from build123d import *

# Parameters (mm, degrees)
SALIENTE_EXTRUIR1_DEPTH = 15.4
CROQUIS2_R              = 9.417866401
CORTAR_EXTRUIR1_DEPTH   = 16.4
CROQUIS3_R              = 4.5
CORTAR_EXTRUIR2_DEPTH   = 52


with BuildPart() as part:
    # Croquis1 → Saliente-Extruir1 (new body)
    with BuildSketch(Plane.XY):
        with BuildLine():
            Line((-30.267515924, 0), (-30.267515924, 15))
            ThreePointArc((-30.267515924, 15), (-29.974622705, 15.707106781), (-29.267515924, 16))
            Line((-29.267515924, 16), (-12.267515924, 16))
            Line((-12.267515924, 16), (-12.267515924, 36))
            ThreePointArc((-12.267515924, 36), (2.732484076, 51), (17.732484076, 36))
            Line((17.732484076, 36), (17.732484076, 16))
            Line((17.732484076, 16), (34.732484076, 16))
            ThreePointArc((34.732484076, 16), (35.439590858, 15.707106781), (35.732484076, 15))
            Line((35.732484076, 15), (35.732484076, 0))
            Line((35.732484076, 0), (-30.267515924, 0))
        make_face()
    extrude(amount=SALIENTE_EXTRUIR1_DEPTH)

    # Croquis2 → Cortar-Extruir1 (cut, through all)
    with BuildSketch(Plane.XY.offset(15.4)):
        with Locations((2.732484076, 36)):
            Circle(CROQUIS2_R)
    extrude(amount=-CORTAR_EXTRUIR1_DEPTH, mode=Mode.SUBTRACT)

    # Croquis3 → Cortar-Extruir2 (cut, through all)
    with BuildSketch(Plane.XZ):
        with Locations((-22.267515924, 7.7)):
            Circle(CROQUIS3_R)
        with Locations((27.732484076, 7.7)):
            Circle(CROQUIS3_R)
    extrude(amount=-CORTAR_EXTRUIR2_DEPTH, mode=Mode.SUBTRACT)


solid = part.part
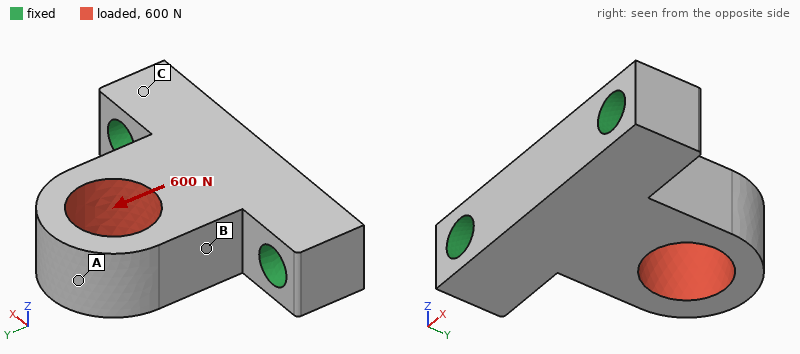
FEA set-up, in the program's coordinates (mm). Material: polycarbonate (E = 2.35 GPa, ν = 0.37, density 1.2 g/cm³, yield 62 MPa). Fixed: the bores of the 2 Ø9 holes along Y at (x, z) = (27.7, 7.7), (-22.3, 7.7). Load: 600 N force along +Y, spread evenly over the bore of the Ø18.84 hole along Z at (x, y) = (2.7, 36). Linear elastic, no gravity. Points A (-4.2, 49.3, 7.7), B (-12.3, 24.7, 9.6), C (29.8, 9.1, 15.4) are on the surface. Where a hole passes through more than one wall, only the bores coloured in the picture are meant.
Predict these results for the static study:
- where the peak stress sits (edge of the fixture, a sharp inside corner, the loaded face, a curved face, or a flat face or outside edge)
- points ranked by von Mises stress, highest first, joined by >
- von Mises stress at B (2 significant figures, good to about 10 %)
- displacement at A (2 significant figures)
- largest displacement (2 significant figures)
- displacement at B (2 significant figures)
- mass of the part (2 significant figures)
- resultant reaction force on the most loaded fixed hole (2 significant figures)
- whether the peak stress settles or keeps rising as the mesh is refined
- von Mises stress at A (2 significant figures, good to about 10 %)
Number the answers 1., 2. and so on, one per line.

1. edge of the fixture
2. B > A > C
3. 2.7 MPa
4. 56 µm
5. 69 µm
6. 31 µm
7. 30 g
8. 310 N
9. keeps rising
10. 1.8 MPa
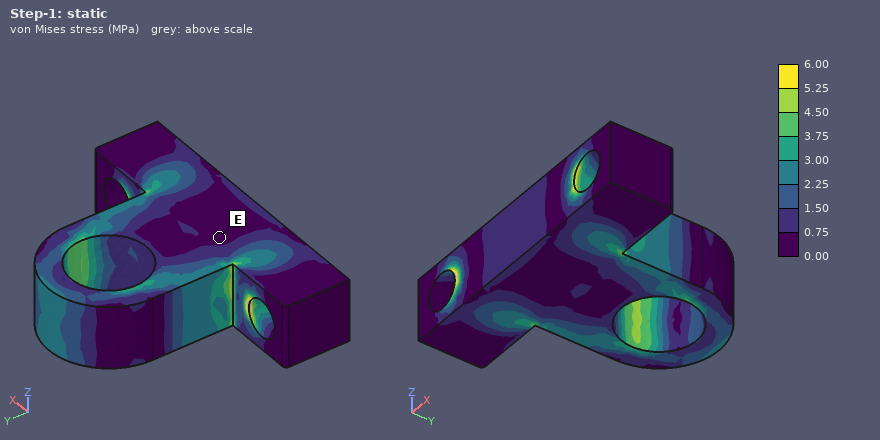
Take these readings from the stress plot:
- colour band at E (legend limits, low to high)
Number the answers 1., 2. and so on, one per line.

1. 0.00 to 0.75 MPa
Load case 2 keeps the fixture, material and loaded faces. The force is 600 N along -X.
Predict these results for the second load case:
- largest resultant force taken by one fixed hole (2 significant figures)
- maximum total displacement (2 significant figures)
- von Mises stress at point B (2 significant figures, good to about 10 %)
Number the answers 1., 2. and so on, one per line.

1. 510 N
2. 0.30 mm
3. 7.5 MPa
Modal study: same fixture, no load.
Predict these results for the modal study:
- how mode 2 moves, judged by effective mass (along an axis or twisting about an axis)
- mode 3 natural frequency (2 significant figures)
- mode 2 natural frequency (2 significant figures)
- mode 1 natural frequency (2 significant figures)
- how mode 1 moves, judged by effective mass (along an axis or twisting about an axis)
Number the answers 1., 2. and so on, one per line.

1. along X
2. 4100 Hz
3. 2800 Hz
4. 1600 Hz
5. along Z
